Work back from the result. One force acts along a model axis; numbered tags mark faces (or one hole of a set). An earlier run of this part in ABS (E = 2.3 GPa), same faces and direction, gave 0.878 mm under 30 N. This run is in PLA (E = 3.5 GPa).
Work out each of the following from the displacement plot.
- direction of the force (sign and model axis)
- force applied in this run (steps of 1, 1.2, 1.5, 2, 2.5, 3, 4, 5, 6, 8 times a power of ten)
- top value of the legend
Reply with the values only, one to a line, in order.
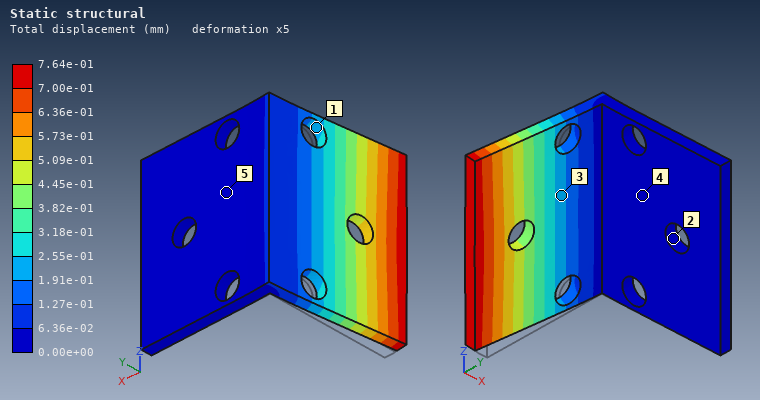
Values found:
-X
40 N
7.64e-01 mm
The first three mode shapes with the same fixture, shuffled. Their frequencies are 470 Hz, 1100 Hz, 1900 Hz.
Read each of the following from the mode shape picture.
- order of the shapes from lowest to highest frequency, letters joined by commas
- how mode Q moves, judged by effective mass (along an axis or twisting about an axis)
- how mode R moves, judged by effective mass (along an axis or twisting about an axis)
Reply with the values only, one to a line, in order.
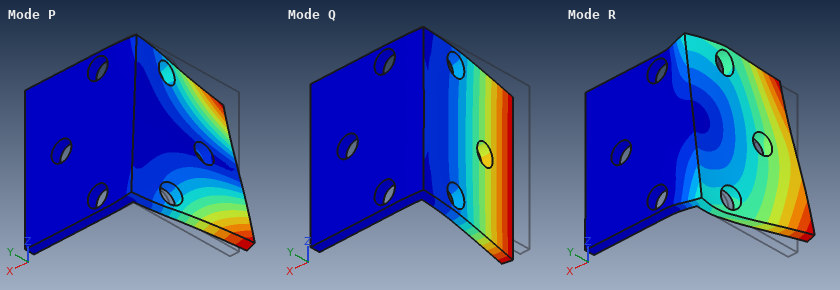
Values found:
Q, P, R
along X
along Z
